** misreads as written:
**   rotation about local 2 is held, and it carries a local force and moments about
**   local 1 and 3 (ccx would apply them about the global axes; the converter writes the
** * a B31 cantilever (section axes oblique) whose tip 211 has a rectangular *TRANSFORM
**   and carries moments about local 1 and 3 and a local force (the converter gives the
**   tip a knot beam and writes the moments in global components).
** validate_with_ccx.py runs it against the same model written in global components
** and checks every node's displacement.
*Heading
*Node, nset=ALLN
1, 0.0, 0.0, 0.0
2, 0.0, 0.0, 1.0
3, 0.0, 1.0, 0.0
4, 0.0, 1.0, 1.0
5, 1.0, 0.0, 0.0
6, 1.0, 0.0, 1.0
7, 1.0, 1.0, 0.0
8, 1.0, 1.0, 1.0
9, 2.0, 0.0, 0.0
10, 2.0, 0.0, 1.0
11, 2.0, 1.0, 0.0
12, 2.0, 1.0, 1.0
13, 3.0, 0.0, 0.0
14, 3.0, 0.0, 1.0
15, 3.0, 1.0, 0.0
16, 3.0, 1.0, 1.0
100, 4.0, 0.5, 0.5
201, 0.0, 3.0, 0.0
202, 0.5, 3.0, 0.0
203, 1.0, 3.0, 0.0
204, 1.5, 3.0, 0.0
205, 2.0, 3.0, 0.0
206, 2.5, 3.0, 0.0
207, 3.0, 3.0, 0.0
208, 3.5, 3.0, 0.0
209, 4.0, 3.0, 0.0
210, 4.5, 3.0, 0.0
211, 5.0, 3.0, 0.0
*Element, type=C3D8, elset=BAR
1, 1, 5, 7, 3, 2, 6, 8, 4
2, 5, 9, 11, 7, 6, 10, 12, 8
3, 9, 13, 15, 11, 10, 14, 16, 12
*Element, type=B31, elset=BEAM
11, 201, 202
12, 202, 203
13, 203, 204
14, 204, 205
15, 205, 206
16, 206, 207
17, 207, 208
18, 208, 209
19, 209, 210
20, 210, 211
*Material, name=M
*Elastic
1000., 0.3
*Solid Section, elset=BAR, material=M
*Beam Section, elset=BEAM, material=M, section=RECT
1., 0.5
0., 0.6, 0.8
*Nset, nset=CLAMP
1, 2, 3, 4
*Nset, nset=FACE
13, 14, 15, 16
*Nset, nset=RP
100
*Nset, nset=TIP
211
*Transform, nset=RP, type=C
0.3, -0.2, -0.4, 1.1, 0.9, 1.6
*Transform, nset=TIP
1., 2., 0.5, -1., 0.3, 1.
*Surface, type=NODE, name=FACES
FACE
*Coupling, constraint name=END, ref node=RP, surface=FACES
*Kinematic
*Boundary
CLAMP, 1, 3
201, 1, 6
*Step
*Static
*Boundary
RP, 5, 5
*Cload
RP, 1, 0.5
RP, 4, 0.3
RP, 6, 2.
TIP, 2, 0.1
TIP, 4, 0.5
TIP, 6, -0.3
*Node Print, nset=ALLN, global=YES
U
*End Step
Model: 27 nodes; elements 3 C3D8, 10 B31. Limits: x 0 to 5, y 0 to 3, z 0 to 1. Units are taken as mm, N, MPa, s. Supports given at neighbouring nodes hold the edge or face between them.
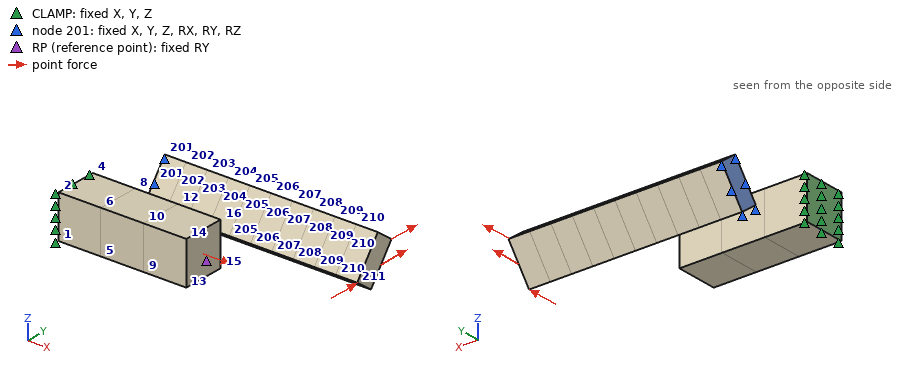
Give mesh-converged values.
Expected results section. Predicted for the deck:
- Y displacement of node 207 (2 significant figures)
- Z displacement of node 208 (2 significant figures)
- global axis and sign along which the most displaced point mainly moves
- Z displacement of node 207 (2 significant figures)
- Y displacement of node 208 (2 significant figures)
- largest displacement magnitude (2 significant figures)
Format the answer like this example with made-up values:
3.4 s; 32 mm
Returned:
-0.069 mm; -0.067 mm; -Y; -0.026 mm; -0.047 mm; 0.23 mm
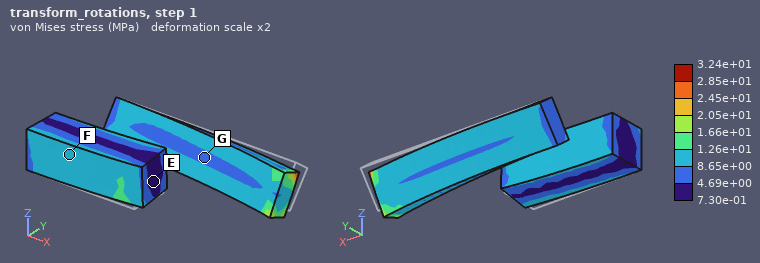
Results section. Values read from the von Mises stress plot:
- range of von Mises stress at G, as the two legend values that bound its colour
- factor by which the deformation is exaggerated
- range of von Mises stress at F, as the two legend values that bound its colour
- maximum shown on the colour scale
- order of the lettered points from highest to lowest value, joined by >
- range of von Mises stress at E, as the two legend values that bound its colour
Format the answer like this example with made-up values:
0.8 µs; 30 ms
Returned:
4.69e+00 to 8.65e+00 MPa; 2; 8.65e+00 to 1.26e+01 MPa; 3.24e+01 MPa; F > G > E; 7.30e-01 to 4.69e+00 MPa
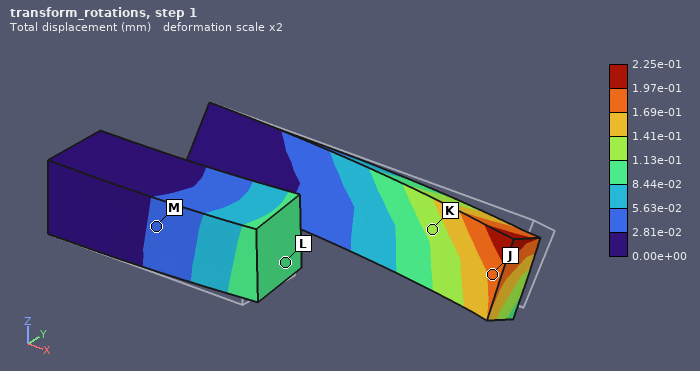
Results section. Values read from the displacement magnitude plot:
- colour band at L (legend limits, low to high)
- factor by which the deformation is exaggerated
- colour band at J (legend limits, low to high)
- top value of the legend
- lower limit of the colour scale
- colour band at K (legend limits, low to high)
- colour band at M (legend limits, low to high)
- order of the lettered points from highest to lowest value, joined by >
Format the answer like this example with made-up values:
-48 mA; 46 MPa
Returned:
8.44e-02 to 1.13e-01 mm; 2; 1.69e-01 to 1.97e-01 mm; 2.25e-01 mm; 0.00e+00 mm; 1.13e-01 to 1.41e-01 mm; 2.81e-02 to 5.63e-02 mm; J > K > L > M
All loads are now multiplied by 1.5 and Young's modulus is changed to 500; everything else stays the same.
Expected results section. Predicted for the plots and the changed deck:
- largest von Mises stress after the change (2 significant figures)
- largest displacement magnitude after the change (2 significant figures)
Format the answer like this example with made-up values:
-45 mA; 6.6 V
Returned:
49 MPa; 0.68 mm
